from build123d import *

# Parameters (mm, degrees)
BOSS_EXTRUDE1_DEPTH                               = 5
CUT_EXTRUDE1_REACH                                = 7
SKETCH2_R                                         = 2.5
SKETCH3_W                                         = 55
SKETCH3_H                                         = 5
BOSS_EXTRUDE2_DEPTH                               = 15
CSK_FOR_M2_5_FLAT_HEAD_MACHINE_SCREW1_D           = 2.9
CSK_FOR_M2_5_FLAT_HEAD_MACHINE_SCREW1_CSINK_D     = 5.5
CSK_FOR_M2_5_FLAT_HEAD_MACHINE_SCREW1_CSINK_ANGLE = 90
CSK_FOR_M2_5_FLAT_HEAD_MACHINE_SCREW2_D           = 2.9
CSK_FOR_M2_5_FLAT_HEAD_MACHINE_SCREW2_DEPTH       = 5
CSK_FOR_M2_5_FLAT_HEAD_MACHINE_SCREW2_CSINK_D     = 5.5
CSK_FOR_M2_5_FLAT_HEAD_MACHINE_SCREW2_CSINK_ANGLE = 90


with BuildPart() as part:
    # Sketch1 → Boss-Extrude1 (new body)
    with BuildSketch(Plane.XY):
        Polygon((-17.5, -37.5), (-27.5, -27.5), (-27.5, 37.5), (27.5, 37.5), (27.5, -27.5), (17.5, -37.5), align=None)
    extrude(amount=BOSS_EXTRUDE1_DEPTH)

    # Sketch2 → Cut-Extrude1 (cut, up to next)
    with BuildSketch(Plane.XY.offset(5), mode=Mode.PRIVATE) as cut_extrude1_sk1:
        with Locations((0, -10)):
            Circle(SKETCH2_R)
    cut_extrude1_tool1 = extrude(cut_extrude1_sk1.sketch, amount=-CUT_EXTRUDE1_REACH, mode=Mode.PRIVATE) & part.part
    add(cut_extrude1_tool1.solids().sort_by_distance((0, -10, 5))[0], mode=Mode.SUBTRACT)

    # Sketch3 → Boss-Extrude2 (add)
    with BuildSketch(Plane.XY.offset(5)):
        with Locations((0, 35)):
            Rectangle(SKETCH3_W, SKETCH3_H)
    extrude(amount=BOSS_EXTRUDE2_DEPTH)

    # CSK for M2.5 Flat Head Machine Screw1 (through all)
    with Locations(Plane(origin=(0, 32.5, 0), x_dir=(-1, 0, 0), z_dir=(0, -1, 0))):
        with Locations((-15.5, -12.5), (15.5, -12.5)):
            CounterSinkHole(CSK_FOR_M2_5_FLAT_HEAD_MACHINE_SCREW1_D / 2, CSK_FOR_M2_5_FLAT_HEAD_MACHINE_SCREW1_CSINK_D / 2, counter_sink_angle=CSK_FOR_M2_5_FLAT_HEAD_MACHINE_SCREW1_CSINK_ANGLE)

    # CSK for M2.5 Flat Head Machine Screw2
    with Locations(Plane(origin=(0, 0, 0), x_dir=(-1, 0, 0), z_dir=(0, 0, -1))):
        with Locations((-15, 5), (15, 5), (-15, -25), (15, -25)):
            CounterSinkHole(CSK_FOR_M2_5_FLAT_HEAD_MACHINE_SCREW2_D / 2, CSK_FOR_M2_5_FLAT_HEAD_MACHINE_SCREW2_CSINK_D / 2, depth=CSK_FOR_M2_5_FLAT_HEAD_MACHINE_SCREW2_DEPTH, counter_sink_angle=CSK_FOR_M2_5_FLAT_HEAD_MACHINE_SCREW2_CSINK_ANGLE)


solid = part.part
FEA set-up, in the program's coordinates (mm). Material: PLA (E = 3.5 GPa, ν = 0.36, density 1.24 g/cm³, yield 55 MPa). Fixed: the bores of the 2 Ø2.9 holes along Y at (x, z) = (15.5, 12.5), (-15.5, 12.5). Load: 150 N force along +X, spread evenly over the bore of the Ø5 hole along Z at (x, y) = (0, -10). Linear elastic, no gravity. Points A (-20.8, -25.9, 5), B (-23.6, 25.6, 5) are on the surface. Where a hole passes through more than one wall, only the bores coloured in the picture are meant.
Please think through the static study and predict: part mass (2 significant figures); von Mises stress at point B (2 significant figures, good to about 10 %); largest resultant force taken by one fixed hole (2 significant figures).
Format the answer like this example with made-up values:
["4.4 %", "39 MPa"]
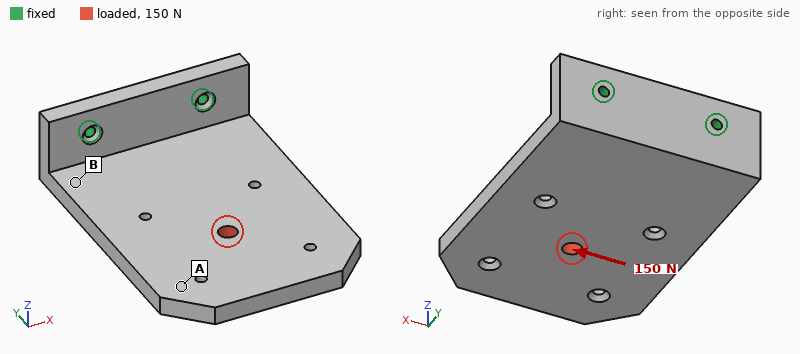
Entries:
["30 g", "5.6 MPa", "220 N"]
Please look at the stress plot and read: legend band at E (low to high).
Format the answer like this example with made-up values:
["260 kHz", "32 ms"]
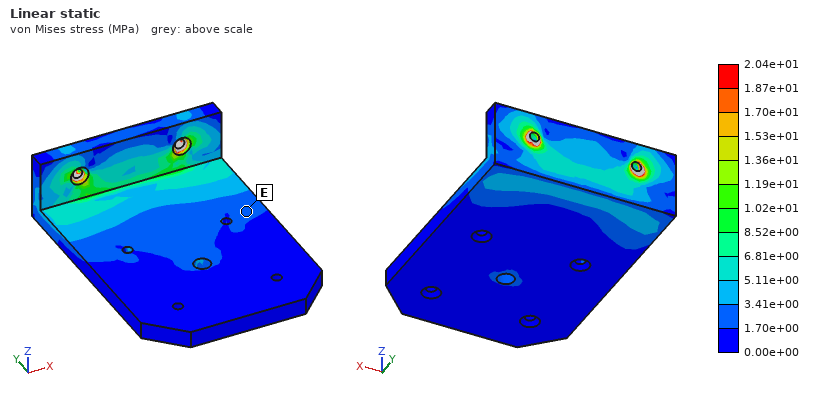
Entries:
["1.70e+00 to 3.41e+00 MPa"]
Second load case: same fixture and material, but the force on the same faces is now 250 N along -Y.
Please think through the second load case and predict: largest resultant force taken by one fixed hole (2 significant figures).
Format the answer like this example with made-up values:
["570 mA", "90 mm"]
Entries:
["130 N"]
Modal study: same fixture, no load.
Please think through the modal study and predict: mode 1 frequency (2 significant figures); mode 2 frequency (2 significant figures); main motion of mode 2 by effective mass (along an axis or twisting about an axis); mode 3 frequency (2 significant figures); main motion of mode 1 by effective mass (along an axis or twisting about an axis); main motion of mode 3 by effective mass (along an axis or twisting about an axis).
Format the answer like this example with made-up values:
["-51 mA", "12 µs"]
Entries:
["200 Hz", "650 Hz", "along X", "880 Hz", "along Z", "along X"]
